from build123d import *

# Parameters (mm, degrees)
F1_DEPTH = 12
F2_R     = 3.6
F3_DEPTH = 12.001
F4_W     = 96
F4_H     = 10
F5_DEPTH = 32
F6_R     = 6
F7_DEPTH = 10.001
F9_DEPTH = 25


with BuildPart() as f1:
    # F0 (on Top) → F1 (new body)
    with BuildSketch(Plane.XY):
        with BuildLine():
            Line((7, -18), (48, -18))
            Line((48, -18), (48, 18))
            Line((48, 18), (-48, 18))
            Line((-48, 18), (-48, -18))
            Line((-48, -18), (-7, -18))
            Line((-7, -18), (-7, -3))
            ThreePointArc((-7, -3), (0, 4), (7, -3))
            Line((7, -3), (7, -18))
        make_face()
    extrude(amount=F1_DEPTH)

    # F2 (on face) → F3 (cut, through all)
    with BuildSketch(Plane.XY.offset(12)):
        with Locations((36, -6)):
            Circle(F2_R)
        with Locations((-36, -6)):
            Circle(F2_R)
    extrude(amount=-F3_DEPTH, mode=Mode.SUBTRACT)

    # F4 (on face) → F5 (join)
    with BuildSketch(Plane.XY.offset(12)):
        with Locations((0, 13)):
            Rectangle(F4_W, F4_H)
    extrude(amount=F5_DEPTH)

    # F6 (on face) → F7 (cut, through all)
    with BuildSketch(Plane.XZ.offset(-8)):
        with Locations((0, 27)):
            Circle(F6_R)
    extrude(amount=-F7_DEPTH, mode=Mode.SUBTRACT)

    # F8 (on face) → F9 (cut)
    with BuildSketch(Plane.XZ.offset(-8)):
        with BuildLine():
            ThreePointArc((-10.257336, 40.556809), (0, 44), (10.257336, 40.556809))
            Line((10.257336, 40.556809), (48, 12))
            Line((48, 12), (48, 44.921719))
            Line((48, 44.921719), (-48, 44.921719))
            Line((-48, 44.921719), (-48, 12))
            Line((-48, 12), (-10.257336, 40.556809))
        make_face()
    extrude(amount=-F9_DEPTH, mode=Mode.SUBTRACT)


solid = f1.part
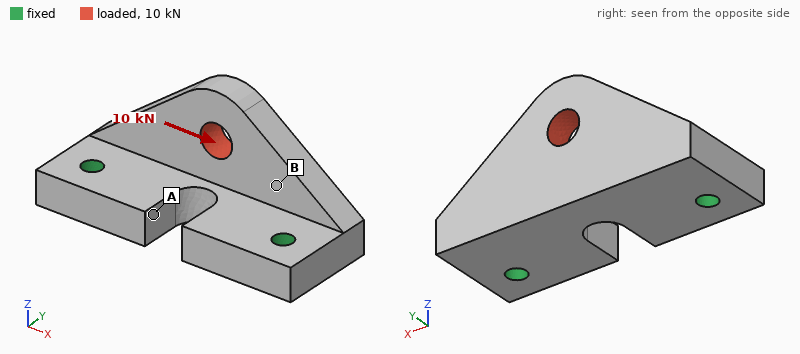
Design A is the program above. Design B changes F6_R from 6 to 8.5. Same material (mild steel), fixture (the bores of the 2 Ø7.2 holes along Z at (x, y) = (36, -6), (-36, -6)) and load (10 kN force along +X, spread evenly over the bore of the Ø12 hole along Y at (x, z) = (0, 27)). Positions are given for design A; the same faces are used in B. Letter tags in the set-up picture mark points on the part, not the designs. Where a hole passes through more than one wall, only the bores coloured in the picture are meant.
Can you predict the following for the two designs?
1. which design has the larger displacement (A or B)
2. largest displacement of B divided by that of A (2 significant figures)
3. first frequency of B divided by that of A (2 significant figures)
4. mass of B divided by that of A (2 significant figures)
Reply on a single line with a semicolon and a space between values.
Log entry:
B; 1.1; 1.0; 0.98
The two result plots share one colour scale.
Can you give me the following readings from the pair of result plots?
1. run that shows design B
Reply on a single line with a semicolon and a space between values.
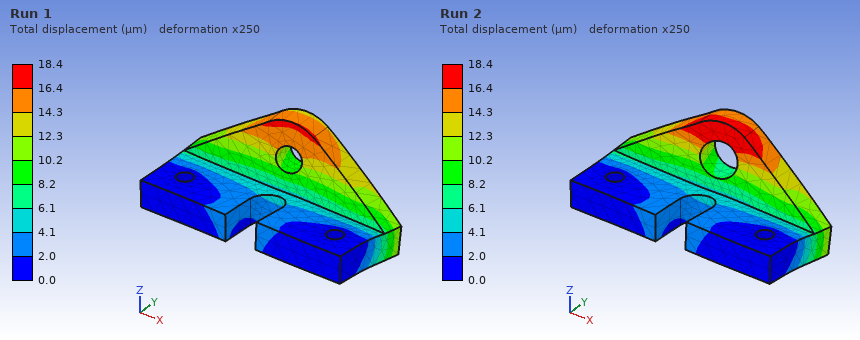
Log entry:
Run 2
